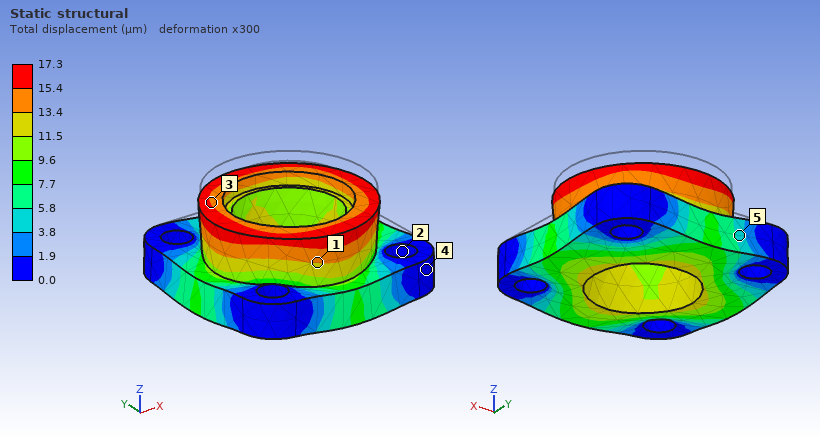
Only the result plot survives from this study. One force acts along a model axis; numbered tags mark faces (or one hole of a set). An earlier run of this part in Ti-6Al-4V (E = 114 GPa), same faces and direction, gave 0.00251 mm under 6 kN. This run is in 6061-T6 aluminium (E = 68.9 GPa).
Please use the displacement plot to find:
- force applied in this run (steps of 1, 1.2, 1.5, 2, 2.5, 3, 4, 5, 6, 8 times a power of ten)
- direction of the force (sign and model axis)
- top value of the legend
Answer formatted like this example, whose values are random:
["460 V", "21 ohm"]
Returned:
["25 kN", "-Z", "17.3 µm"]
